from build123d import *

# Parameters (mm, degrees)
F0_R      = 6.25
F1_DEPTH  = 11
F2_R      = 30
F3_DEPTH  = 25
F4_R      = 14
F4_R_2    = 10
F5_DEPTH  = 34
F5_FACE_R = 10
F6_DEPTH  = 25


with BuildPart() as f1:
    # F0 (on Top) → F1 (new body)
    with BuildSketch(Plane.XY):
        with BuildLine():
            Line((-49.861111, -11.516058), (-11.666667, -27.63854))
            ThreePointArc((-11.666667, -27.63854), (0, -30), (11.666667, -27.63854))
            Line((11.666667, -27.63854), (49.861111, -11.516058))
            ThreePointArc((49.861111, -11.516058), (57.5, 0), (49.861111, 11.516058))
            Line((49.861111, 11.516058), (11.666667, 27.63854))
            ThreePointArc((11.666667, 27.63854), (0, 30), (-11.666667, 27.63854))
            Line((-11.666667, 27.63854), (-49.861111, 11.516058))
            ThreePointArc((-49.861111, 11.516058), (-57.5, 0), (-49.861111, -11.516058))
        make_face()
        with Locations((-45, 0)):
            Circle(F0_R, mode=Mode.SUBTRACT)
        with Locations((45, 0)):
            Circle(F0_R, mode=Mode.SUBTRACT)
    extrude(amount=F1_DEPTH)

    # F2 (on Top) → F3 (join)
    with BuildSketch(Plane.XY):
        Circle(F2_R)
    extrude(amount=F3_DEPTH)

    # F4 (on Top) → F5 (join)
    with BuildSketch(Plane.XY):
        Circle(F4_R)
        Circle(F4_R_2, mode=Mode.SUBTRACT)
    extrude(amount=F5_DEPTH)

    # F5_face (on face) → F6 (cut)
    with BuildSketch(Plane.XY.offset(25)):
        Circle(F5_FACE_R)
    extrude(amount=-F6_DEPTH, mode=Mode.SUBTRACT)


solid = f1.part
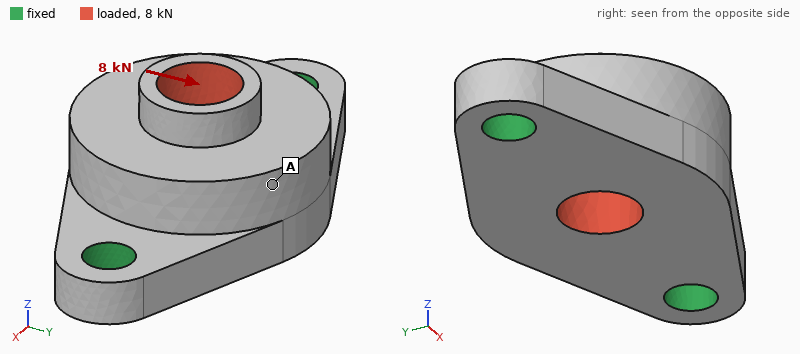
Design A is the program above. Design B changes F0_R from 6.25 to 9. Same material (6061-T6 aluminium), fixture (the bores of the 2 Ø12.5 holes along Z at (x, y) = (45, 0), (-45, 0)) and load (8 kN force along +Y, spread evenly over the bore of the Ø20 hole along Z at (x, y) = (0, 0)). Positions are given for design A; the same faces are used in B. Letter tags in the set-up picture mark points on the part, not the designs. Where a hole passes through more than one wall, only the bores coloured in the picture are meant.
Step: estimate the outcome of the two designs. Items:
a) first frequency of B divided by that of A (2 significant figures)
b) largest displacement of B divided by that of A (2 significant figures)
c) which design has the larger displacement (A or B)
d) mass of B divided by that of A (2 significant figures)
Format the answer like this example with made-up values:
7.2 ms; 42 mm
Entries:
1.2; 0.74; A; 0.96
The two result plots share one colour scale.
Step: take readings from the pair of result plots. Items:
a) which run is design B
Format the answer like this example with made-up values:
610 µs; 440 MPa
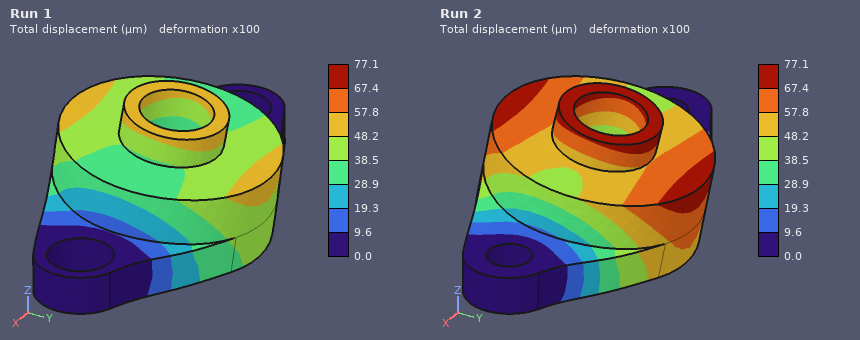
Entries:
Run 1
